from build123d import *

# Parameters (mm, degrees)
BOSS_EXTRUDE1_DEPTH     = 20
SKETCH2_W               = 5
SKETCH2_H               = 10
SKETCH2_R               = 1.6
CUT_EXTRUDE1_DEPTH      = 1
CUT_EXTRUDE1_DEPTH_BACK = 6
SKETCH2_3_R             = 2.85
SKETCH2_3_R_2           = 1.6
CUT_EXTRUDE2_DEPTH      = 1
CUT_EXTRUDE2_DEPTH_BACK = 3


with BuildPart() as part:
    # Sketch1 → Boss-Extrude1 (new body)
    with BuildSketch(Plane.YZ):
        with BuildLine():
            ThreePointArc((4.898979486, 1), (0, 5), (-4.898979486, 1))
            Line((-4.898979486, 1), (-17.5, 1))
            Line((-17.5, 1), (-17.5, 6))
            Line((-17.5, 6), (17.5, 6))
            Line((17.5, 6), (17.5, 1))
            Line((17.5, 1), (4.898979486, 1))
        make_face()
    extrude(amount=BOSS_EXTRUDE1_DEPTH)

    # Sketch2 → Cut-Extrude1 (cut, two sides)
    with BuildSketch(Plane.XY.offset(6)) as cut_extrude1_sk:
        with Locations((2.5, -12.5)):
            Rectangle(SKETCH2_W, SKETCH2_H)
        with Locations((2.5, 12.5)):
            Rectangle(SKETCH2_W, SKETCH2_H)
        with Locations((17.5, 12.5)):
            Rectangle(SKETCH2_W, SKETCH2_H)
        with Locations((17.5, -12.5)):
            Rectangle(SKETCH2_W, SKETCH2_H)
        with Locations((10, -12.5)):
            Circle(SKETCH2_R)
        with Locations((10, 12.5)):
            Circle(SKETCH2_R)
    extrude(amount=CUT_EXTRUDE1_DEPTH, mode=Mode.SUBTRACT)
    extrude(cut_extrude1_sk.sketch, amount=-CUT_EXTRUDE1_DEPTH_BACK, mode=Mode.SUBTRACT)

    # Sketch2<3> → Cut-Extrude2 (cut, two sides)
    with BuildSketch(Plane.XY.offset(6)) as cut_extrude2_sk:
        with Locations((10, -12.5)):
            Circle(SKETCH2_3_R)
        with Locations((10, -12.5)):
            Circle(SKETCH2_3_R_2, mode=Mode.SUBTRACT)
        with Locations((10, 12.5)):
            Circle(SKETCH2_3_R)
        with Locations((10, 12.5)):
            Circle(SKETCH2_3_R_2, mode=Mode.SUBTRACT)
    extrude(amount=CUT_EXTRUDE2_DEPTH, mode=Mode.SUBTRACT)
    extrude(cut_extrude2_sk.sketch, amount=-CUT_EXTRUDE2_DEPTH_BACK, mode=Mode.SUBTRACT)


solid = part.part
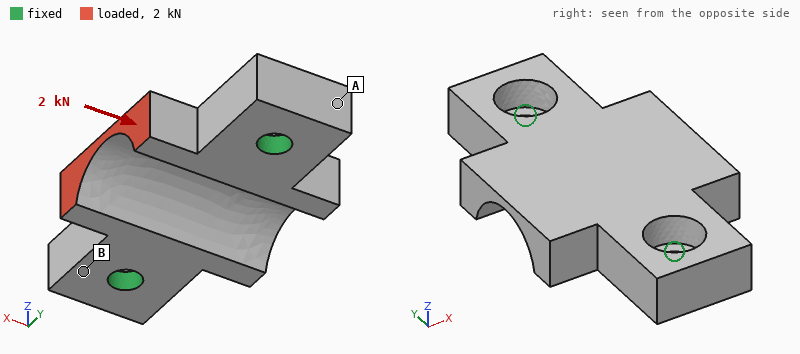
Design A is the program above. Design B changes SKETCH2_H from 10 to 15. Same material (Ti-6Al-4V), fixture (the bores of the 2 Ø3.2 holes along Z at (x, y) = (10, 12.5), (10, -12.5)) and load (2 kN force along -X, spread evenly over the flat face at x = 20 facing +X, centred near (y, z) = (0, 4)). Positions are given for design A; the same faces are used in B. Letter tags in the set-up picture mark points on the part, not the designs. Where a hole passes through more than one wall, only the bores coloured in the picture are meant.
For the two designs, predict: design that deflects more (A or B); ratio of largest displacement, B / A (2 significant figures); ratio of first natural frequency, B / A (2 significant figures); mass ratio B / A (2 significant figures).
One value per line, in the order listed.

B
1.5
1.2
0.86
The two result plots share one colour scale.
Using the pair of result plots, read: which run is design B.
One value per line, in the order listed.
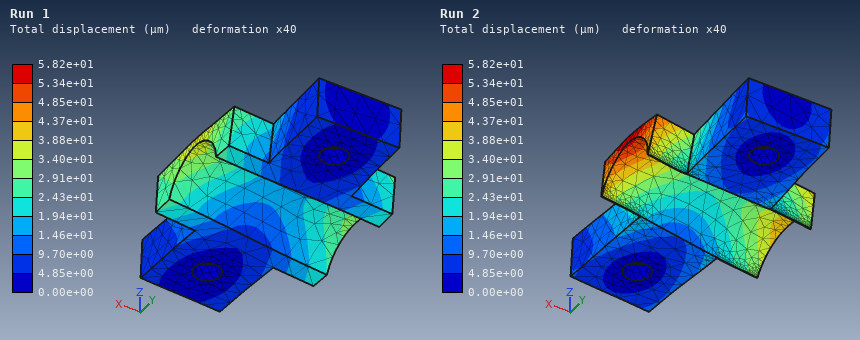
Run 2
